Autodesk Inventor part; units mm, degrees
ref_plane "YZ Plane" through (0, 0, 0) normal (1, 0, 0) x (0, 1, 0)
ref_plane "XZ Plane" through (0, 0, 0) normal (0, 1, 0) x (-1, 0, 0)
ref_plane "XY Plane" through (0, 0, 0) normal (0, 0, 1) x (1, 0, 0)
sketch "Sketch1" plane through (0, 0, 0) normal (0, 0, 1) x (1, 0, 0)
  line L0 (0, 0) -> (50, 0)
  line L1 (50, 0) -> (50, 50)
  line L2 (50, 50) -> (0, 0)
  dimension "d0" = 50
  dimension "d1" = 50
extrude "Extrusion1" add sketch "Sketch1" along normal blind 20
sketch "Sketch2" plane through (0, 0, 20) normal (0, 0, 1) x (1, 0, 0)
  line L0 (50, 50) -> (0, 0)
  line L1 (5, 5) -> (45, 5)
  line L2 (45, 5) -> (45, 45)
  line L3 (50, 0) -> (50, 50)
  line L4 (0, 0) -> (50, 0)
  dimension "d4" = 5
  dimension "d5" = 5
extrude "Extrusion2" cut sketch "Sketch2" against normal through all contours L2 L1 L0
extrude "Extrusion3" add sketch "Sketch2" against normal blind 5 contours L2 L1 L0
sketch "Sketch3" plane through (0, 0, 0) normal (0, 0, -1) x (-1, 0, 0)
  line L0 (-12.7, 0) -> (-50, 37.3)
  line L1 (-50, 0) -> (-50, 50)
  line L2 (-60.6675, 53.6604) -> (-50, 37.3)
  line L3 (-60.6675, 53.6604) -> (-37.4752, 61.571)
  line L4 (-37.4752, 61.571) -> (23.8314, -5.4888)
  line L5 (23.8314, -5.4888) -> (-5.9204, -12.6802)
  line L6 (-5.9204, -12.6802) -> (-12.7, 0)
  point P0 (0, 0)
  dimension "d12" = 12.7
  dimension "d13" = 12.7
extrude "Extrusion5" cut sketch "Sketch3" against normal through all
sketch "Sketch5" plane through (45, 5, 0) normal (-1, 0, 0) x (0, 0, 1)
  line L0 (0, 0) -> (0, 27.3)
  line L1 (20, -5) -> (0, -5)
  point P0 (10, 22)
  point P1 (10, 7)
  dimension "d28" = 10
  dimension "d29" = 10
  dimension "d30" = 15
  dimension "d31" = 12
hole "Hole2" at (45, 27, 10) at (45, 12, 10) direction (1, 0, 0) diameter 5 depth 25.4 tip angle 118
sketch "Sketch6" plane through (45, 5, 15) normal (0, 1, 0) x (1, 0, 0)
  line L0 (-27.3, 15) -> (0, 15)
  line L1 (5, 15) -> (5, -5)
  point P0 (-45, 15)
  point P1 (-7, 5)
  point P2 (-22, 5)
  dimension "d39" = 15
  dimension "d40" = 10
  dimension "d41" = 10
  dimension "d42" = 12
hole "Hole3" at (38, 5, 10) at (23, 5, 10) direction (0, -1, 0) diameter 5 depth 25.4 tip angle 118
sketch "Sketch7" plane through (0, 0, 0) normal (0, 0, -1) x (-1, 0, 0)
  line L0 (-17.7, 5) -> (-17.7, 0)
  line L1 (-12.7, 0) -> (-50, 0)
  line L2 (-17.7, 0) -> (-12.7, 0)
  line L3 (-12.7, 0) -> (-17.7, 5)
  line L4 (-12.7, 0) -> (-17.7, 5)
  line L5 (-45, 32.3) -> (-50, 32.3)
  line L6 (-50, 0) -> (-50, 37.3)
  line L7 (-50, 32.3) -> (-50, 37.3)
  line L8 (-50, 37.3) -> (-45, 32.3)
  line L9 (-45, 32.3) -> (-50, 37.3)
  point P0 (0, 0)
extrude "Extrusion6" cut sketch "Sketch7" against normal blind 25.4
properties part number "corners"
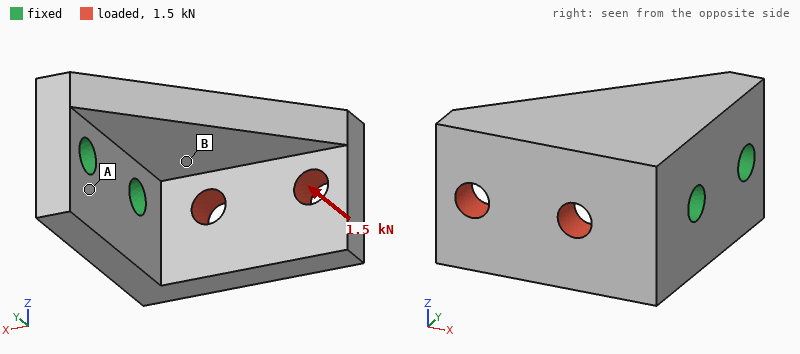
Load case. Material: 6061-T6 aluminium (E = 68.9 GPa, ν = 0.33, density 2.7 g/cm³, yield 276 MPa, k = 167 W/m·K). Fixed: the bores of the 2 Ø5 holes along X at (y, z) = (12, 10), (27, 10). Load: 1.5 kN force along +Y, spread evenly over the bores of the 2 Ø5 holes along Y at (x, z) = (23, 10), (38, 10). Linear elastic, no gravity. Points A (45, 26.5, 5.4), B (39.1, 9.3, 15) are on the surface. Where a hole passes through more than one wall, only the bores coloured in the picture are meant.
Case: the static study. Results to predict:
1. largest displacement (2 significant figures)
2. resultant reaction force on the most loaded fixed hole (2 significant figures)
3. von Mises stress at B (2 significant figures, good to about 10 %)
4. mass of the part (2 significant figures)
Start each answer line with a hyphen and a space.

- 0.17 mm
- 1.5 kN
- 43 MPa
- 20 g
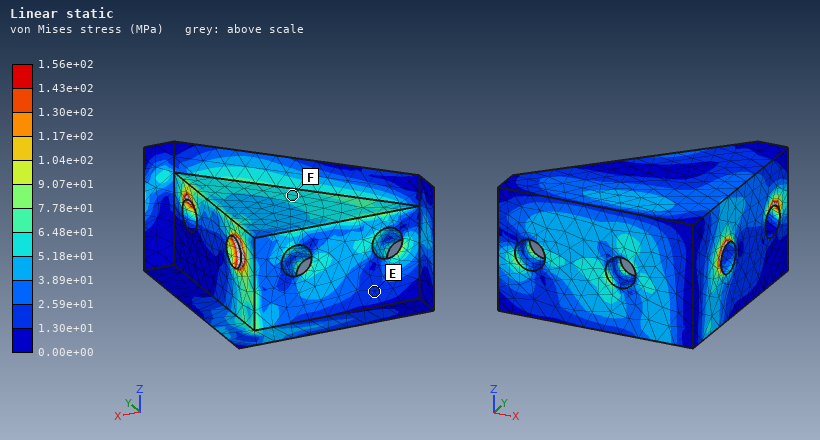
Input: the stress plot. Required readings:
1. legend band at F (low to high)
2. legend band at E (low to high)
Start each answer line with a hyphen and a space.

- 5.18e+01 to 6.48e+01 MPa
- 1.30e+01 to 2.59e+01 MPa
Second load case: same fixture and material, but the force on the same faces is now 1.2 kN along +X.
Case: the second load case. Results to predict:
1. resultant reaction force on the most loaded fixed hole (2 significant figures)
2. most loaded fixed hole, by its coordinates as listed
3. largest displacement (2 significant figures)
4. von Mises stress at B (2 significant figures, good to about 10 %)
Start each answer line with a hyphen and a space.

- 1.5 kN
- (12, 10)
- 38 µm
- 16 MPa
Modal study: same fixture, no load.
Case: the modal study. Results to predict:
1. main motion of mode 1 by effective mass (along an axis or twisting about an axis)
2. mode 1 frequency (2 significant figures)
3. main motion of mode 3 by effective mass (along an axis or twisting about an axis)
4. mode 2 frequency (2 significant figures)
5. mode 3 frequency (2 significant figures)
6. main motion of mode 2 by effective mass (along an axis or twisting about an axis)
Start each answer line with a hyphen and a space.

- along Z
- 5300 Hz
- along X
- 7600 Hz
- 14 kHz
- along Y
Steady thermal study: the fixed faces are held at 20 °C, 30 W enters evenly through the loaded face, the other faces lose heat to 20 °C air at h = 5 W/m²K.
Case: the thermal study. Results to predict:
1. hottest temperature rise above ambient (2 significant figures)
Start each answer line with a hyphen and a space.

- 33 K
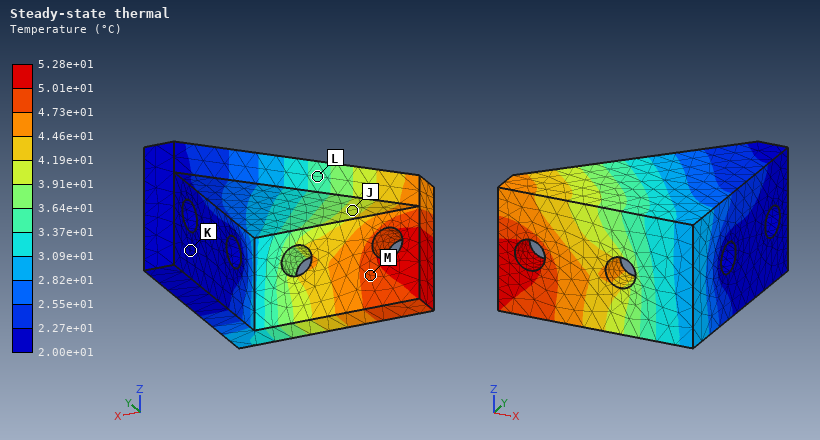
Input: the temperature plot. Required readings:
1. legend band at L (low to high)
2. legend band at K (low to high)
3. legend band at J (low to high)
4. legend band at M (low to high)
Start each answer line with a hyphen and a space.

- 3.37e+01 to 3.64e+01 °C
- 2.00e+01 to 2.27e+01 °C
- 3.91e+01 to 4.19e+01 °C
- 4.73e+01 to 5.01e+01 °C
